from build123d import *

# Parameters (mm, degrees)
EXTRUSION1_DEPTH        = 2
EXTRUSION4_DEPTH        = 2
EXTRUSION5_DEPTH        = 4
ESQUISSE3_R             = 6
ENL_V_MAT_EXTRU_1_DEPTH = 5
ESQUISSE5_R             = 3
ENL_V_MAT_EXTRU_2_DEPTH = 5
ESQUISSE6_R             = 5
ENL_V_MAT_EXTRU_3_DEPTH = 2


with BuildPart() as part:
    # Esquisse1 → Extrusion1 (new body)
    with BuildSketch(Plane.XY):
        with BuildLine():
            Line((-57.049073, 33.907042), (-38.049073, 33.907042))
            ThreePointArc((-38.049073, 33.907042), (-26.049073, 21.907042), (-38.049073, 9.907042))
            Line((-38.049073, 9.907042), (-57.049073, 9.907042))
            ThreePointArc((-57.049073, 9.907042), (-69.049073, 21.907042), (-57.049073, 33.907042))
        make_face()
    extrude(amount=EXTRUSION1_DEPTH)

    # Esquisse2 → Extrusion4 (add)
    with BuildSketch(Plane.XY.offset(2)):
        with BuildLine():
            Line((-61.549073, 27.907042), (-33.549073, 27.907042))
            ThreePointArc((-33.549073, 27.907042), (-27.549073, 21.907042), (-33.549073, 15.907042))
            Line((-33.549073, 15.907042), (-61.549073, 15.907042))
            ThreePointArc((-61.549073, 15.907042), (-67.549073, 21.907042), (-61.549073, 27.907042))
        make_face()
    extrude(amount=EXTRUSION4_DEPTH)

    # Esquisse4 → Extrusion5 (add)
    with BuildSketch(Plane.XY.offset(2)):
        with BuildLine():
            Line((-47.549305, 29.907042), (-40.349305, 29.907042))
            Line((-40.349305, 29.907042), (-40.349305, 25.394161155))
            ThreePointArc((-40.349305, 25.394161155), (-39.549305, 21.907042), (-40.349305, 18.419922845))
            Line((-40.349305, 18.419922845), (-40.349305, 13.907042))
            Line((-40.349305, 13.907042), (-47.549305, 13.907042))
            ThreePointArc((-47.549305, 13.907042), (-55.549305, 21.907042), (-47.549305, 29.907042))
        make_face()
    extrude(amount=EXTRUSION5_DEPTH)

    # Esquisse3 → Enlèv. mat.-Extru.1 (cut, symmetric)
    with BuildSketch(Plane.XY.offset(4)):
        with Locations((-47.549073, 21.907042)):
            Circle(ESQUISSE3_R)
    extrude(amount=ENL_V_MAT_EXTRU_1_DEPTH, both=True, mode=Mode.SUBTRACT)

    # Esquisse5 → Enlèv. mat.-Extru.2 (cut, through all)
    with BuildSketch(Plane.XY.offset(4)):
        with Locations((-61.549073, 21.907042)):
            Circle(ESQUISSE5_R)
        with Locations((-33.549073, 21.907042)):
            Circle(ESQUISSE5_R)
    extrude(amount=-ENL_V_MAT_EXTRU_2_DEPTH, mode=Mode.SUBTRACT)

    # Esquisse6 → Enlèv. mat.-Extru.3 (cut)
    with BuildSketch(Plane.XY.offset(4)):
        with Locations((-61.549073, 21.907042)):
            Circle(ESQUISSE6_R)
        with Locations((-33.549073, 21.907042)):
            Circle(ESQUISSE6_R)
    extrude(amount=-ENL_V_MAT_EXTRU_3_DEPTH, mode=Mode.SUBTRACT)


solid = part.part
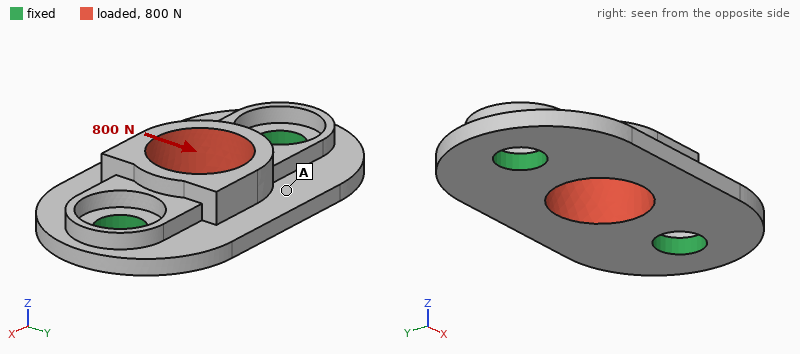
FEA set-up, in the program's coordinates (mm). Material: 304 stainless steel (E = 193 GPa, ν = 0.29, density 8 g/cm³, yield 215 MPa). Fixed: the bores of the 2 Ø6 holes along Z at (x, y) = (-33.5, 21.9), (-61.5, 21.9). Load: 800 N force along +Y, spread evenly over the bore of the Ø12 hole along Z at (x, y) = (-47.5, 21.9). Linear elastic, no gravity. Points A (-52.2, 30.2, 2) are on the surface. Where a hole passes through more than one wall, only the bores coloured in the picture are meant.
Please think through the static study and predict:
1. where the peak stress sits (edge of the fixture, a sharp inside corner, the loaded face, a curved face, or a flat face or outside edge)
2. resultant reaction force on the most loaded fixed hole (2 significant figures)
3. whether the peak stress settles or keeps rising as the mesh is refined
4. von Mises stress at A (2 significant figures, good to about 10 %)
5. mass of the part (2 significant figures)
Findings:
edge of the fixture
400 N
keeps rising
12 MPa
17 g
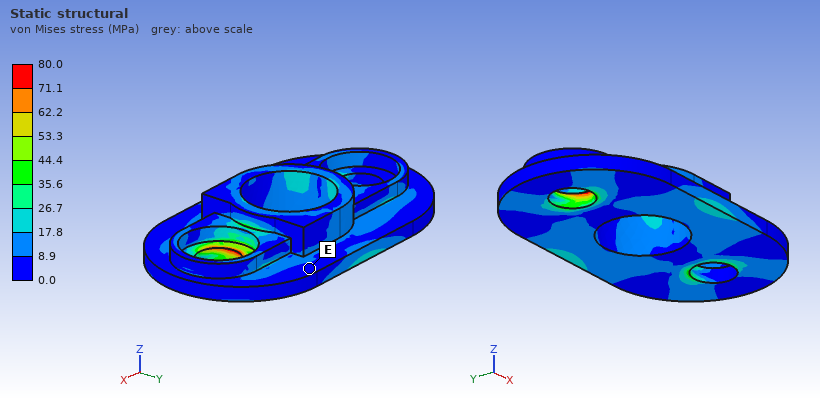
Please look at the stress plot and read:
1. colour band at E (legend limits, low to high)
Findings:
0.0 to 8.9 MPa
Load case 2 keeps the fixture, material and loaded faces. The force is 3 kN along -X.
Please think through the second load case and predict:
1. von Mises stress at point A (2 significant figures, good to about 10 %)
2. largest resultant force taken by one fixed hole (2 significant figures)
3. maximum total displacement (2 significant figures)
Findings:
14 MPa
1.5 kN
3.6 µm
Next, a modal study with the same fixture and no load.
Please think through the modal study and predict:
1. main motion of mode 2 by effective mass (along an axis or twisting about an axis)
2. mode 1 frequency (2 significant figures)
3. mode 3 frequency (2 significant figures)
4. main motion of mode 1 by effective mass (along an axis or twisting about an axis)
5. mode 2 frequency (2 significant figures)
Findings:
along Z
13 kHz
26 kHz
twisting about X
17 kHz
